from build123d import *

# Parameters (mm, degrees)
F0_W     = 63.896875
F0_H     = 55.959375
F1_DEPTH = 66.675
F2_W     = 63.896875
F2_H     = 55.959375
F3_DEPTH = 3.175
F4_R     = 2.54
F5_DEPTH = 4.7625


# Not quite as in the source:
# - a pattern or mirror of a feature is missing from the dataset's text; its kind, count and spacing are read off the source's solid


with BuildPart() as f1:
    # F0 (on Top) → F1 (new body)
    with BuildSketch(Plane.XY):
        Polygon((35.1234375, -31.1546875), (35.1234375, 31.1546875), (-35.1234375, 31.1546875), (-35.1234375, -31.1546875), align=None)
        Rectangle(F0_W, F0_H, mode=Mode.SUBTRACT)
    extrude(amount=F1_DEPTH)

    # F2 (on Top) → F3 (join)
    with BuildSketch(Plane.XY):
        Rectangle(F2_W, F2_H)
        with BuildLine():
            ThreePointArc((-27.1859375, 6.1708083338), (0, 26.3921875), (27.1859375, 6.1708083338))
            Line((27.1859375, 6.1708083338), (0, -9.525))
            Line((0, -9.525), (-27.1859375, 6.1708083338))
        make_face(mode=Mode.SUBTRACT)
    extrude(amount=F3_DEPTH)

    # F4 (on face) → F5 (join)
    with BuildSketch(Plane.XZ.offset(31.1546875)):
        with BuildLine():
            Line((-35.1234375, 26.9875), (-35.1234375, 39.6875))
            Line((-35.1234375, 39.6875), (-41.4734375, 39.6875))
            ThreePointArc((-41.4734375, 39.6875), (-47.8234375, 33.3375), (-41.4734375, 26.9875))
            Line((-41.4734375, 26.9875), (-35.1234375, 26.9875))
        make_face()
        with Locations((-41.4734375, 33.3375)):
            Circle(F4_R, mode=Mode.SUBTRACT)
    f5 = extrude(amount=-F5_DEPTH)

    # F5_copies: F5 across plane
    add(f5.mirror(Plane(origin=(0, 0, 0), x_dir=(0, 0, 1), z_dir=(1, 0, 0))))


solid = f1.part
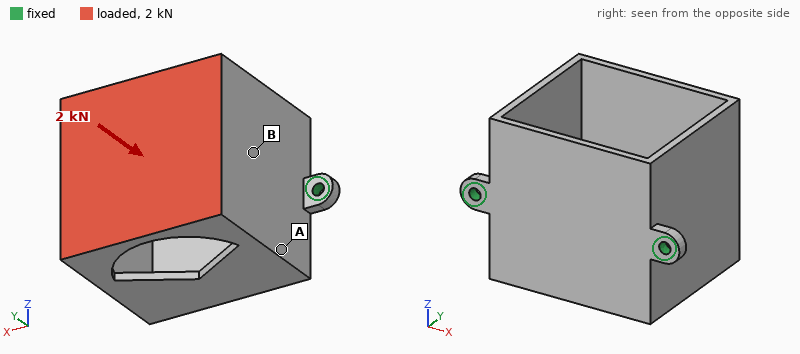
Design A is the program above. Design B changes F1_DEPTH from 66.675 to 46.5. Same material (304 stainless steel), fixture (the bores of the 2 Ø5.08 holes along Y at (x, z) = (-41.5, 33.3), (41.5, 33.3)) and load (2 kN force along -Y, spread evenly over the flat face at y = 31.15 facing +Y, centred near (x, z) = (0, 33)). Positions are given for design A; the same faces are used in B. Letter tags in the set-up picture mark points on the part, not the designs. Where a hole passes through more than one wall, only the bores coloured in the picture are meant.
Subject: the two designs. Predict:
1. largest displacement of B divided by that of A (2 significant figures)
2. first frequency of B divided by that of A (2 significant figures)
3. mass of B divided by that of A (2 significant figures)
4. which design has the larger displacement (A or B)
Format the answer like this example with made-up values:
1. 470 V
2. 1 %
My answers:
1. 1.5
2. 1.2
3. 0.74
4. B
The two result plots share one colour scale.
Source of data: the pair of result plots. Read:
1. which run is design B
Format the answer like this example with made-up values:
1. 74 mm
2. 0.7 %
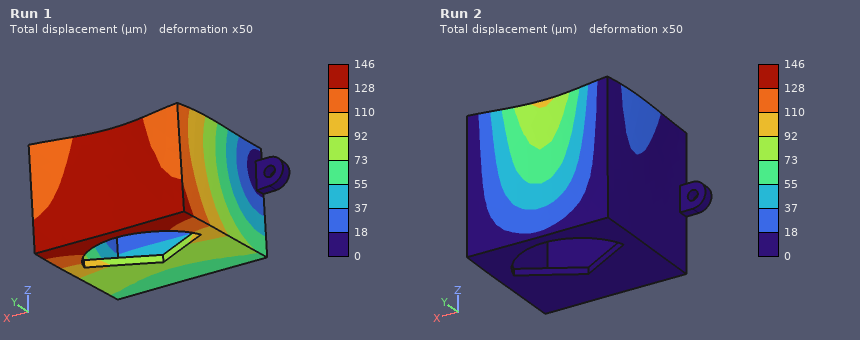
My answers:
1. Run 1
